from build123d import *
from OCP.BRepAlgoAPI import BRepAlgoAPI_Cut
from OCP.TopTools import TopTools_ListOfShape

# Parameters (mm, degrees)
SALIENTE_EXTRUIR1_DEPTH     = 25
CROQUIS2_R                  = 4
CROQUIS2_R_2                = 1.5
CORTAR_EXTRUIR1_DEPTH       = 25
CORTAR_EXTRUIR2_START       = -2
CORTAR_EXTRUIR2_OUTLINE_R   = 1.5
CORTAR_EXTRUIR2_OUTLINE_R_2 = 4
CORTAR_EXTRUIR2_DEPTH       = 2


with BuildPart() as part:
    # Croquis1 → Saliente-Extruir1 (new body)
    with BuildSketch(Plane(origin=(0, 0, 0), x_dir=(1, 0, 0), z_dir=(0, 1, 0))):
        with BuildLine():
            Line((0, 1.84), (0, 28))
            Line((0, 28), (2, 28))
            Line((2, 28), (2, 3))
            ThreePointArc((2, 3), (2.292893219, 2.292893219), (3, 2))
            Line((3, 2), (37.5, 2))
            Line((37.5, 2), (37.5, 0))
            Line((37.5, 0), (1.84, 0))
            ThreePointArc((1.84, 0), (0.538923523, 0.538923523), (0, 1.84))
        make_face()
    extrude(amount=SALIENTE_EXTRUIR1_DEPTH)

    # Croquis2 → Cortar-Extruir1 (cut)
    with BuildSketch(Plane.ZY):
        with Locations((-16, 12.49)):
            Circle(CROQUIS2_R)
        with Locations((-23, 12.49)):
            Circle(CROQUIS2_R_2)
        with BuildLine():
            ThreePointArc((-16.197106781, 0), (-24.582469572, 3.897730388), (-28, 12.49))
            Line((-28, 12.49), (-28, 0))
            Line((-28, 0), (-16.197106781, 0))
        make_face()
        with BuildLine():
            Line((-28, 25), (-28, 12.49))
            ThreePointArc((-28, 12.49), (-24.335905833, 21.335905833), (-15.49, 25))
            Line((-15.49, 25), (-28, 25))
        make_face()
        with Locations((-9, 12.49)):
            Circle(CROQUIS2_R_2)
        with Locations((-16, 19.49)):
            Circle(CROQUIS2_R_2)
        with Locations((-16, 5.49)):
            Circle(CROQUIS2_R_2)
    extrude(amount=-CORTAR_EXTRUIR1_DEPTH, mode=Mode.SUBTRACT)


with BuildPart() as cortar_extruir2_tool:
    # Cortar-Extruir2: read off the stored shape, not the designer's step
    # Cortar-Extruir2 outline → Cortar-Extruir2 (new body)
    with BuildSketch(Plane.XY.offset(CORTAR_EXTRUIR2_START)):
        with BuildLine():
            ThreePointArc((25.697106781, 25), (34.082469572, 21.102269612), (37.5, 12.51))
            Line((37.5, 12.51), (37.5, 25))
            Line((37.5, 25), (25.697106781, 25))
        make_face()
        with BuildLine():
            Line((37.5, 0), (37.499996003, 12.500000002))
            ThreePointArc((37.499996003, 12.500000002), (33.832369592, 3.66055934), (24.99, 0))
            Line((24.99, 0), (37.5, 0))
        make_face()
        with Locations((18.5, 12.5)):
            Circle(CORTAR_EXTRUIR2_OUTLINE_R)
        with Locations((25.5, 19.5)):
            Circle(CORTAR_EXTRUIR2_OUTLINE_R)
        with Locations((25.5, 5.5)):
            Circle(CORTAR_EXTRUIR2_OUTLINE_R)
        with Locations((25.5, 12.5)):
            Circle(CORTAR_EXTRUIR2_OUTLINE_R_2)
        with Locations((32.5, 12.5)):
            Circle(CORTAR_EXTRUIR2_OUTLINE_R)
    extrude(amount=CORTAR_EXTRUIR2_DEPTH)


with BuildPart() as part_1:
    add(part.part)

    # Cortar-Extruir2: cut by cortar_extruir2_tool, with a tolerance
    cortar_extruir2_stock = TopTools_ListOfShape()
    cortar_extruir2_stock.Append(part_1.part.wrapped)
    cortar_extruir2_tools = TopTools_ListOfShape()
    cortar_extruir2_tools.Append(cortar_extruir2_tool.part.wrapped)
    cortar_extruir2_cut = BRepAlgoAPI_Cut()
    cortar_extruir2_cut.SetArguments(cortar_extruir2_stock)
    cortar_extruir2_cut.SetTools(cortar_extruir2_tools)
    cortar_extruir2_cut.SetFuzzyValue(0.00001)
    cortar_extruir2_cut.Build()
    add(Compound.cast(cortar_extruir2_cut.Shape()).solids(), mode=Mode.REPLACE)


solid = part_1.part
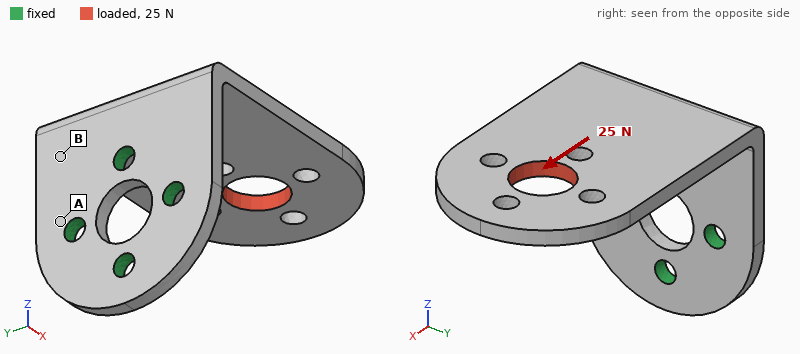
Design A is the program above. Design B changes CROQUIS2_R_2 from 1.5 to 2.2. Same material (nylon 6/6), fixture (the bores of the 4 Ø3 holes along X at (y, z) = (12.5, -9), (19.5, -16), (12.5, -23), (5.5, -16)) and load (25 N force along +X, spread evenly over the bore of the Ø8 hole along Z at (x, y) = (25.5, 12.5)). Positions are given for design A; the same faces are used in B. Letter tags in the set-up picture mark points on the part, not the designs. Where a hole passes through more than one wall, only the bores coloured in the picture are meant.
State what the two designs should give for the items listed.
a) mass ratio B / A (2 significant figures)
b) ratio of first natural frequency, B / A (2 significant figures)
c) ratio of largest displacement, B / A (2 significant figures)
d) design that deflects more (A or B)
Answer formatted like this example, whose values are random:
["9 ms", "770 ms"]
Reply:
["0.97", "1.0", "0.79", "A"]
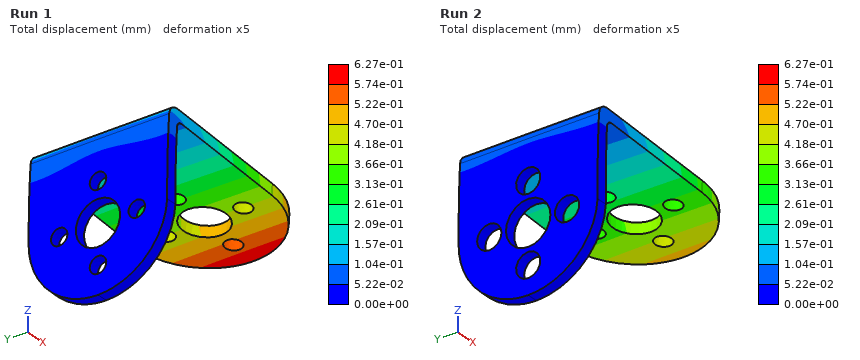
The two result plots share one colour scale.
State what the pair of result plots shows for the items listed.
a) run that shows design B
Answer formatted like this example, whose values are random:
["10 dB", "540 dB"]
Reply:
["Run 2"]
